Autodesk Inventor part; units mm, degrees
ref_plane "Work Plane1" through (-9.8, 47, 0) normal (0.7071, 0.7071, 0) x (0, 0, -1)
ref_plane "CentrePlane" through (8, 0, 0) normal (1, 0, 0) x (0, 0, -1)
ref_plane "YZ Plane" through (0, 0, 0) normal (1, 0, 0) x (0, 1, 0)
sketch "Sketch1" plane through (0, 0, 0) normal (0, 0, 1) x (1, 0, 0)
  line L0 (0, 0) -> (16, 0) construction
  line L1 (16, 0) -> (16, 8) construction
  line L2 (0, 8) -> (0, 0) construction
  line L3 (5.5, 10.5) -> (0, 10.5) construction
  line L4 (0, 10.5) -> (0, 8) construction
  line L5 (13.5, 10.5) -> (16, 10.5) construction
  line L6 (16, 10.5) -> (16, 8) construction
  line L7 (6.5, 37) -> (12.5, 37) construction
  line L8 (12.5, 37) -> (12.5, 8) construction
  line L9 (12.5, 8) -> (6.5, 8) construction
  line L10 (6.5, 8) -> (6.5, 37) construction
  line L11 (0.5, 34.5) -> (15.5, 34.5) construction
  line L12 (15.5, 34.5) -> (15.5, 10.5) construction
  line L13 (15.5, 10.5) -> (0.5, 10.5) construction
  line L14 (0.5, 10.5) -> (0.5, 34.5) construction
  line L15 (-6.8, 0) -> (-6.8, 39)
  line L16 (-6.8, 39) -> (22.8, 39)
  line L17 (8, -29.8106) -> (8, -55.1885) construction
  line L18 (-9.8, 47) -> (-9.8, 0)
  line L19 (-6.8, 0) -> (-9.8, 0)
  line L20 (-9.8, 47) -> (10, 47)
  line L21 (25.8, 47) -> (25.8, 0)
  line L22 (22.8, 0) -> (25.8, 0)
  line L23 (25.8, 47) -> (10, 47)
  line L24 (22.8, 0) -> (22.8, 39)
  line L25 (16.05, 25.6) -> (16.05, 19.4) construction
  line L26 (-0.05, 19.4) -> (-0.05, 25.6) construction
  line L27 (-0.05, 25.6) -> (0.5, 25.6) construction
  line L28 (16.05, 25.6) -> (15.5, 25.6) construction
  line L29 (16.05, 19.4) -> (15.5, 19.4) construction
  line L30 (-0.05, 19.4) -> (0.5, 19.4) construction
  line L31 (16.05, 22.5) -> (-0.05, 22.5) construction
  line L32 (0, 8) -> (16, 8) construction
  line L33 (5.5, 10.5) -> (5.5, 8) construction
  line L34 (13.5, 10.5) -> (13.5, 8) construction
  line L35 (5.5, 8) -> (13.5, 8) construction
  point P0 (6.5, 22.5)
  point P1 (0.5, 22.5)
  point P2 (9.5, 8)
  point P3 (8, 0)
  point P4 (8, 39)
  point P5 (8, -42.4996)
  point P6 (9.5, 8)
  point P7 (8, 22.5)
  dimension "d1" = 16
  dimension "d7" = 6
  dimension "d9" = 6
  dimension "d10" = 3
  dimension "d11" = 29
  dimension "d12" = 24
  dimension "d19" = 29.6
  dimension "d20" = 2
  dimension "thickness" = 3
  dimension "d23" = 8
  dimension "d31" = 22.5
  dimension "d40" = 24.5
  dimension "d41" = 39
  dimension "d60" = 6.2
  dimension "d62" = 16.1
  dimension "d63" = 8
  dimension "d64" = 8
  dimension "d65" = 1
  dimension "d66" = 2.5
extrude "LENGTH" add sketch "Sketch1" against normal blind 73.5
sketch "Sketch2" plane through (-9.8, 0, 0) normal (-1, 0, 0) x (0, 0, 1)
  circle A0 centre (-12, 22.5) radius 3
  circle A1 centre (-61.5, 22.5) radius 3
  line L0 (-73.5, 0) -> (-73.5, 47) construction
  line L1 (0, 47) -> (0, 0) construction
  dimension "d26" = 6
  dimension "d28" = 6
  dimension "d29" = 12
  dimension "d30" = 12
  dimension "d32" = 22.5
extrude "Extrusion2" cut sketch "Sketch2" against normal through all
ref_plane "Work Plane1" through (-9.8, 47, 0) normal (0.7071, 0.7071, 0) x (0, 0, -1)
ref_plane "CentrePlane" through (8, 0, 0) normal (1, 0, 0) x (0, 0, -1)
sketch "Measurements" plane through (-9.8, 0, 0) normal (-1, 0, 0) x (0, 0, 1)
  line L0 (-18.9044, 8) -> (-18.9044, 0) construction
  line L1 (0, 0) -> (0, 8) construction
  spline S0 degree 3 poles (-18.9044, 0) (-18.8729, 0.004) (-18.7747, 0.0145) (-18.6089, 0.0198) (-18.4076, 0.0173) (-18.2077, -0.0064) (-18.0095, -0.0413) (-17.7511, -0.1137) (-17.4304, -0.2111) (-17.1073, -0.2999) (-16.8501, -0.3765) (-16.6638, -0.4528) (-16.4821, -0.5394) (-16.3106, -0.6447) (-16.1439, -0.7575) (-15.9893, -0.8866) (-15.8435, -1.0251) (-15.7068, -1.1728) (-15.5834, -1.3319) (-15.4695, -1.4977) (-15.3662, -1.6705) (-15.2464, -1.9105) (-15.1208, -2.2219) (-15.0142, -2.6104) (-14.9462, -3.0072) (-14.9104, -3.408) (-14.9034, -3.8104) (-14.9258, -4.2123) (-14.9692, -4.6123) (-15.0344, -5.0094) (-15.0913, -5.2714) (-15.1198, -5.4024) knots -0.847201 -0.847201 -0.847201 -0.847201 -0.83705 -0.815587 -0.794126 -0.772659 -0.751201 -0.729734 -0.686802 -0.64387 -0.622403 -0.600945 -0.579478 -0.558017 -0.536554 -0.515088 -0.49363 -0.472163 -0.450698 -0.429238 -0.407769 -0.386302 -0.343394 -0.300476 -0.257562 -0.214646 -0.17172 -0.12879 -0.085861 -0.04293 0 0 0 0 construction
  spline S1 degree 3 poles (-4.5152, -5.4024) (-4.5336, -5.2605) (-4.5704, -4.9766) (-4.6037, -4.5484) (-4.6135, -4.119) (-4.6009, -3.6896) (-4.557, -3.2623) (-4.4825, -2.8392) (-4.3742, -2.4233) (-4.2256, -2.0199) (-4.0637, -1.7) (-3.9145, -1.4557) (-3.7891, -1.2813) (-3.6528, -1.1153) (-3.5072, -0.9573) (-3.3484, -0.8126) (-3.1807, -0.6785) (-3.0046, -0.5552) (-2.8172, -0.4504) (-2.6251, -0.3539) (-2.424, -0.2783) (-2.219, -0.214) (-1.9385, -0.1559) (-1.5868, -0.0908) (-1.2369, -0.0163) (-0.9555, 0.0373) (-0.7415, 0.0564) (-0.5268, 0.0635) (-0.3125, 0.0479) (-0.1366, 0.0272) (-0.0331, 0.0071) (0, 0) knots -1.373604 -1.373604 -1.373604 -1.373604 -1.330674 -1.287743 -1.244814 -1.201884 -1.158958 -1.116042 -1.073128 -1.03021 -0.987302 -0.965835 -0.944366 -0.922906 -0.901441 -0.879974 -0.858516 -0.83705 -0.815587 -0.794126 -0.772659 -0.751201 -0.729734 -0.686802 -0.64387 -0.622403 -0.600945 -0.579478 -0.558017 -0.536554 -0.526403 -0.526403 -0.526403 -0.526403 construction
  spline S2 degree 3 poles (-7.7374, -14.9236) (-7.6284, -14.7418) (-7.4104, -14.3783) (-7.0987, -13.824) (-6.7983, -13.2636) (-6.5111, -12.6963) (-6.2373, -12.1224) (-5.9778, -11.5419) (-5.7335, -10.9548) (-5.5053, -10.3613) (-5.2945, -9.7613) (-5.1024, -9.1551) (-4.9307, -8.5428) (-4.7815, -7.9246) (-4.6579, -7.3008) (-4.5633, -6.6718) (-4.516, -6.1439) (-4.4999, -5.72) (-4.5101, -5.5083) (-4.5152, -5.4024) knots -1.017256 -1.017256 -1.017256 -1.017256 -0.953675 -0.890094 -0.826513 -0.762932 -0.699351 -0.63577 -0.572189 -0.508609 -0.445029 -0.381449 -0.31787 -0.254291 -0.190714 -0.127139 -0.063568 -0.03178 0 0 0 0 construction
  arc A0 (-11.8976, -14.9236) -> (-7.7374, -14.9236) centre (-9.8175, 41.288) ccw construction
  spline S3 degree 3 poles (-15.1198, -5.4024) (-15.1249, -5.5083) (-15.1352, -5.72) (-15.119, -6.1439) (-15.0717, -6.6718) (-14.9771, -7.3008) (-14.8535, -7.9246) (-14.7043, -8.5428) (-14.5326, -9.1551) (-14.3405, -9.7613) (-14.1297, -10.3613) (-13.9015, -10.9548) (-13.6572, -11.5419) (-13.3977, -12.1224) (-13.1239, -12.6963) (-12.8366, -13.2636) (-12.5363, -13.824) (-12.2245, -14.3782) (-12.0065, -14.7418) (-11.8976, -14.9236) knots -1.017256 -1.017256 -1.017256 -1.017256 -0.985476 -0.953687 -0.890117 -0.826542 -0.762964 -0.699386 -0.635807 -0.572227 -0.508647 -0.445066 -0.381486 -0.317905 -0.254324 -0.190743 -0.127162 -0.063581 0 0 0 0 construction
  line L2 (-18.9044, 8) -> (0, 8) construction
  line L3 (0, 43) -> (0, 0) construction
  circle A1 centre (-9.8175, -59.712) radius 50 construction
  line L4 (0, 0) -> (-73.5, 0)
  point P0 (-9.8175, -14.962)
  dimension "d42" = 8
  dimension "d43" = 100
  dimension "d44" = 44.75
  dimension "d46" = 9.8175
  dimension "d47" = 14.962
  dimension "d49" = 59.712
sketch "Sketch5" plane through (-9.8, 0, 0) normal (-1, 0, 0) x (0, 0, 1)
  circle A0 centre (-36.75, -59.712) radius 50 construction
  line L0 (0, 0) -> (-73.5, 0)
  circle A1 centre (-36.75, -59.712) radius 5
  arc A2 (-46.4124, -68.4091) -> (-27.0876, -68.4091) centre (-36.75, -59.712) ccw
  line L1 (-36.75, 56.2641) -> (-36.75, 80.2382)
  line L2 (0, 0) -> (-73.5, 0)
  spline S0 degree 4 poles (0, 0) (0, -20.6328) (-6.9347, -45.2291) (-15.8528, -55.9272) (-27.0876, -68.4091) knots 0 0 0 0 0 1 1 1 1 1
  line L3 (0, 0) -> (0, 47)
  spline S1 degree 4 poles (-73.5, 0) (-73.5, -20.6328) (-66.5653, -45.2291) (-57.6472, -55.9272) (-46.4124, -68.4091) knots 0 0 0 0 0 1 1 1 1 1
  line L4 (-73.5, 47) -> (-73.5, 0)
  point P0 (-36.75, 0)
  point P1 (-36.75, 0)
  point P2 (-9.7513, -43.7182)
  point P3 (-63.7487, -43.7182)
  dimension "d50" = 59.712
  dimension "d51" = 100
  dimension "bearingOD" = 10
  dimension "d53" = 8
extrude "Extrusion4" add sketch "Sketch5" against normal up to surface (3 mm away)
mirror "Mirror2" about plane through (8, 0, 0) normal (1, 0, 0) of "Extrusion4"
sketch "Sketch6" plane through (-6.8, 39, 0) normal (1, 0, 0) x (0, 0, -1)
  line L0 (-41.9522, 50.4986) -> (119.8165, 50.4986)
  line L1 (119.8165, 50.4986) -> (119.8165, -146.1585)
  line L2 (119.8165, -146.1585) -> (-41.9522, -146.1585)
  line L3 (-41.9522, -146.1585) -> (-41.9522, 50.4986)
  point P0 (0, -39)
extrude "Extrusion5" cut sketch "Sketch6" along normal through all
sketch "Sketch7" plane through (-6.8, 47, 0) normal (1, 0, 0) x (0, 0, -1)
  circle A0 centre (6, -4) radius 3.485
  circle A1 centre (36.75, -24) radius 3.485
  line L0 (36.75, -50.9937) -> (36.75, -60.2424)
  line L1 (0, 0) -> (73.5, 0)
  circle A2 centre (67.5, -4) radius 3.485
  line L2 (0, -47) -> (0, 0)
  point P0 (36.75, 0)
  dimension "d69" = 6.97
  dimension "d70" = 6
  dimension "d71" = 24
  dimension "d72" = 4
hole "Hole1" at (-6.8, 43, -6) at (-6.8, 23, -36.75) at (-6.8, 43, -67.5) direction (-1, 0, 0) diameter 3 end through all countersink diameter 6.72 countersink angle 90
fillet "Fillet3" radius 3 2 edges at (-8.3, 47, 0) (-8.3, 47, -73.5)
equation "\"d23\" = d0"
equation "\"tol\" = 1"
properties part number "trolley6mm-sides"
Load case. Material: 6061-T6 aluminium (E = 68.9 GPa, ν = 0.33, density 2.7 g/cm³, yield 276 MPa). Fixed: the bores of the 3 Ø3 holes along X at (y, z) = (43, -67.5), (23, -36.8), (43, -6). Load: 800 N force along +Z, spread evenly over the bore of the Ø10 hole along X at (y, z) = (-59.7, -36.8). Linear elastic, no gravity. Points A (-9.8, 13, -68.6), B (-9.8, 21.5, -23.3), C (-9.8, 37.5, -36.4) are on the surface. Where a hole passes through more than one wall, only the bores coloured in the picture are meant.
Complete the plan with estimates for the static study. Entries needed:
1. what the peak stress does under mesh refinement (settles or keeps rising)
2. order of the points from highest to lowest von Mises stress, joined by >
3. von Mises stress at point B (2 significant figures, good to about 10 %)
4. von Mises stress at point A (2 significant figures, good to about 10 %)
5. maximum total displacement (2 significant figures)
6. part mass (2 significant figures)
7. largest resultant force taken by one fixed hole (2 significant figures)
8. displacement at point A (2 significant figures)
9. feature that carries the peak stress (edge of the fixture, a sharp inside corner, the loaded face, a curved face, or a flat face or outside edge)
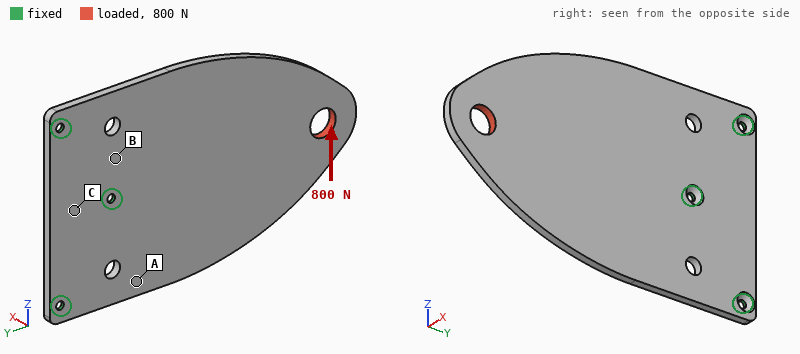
keeps rising
A > B > C
12 MPa
23 MPa
86 µm
58 g
1.0 kN
26 µm
edge of the fixture
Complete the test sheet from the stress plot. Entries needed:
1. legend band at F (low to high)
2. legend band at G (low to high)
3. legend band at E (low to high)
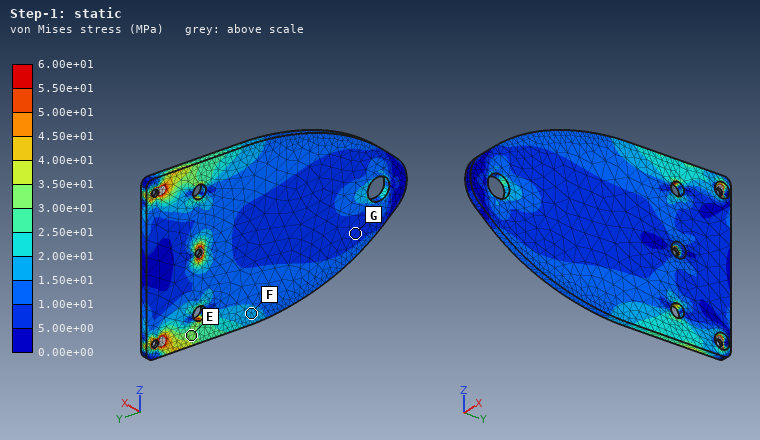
1.50e+01 to 2.00e+01 MPa
5.00e+00 to 1.00e+01 MPa
3.00e+01 to 3.50e+01 MPa
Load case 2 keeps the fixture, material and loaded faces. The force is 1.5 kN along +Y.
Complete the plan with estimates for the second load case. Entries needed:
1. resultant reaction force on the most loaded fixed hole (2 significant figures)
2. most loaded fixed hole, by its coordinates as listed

740 N
(23, -36.8)
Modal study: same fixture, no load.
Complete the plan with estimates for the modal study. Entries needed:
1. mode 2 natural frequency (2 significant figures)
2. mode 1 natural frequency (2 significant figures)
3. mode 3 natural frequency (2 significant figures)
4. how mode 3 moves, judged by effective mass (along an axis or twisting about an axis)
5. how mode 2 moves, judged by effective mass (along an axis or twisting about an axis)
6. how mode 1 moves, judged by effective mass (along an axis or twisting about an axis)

930 Hz
310 Hz
1500 Hz
along X
twisting about Y
along X
